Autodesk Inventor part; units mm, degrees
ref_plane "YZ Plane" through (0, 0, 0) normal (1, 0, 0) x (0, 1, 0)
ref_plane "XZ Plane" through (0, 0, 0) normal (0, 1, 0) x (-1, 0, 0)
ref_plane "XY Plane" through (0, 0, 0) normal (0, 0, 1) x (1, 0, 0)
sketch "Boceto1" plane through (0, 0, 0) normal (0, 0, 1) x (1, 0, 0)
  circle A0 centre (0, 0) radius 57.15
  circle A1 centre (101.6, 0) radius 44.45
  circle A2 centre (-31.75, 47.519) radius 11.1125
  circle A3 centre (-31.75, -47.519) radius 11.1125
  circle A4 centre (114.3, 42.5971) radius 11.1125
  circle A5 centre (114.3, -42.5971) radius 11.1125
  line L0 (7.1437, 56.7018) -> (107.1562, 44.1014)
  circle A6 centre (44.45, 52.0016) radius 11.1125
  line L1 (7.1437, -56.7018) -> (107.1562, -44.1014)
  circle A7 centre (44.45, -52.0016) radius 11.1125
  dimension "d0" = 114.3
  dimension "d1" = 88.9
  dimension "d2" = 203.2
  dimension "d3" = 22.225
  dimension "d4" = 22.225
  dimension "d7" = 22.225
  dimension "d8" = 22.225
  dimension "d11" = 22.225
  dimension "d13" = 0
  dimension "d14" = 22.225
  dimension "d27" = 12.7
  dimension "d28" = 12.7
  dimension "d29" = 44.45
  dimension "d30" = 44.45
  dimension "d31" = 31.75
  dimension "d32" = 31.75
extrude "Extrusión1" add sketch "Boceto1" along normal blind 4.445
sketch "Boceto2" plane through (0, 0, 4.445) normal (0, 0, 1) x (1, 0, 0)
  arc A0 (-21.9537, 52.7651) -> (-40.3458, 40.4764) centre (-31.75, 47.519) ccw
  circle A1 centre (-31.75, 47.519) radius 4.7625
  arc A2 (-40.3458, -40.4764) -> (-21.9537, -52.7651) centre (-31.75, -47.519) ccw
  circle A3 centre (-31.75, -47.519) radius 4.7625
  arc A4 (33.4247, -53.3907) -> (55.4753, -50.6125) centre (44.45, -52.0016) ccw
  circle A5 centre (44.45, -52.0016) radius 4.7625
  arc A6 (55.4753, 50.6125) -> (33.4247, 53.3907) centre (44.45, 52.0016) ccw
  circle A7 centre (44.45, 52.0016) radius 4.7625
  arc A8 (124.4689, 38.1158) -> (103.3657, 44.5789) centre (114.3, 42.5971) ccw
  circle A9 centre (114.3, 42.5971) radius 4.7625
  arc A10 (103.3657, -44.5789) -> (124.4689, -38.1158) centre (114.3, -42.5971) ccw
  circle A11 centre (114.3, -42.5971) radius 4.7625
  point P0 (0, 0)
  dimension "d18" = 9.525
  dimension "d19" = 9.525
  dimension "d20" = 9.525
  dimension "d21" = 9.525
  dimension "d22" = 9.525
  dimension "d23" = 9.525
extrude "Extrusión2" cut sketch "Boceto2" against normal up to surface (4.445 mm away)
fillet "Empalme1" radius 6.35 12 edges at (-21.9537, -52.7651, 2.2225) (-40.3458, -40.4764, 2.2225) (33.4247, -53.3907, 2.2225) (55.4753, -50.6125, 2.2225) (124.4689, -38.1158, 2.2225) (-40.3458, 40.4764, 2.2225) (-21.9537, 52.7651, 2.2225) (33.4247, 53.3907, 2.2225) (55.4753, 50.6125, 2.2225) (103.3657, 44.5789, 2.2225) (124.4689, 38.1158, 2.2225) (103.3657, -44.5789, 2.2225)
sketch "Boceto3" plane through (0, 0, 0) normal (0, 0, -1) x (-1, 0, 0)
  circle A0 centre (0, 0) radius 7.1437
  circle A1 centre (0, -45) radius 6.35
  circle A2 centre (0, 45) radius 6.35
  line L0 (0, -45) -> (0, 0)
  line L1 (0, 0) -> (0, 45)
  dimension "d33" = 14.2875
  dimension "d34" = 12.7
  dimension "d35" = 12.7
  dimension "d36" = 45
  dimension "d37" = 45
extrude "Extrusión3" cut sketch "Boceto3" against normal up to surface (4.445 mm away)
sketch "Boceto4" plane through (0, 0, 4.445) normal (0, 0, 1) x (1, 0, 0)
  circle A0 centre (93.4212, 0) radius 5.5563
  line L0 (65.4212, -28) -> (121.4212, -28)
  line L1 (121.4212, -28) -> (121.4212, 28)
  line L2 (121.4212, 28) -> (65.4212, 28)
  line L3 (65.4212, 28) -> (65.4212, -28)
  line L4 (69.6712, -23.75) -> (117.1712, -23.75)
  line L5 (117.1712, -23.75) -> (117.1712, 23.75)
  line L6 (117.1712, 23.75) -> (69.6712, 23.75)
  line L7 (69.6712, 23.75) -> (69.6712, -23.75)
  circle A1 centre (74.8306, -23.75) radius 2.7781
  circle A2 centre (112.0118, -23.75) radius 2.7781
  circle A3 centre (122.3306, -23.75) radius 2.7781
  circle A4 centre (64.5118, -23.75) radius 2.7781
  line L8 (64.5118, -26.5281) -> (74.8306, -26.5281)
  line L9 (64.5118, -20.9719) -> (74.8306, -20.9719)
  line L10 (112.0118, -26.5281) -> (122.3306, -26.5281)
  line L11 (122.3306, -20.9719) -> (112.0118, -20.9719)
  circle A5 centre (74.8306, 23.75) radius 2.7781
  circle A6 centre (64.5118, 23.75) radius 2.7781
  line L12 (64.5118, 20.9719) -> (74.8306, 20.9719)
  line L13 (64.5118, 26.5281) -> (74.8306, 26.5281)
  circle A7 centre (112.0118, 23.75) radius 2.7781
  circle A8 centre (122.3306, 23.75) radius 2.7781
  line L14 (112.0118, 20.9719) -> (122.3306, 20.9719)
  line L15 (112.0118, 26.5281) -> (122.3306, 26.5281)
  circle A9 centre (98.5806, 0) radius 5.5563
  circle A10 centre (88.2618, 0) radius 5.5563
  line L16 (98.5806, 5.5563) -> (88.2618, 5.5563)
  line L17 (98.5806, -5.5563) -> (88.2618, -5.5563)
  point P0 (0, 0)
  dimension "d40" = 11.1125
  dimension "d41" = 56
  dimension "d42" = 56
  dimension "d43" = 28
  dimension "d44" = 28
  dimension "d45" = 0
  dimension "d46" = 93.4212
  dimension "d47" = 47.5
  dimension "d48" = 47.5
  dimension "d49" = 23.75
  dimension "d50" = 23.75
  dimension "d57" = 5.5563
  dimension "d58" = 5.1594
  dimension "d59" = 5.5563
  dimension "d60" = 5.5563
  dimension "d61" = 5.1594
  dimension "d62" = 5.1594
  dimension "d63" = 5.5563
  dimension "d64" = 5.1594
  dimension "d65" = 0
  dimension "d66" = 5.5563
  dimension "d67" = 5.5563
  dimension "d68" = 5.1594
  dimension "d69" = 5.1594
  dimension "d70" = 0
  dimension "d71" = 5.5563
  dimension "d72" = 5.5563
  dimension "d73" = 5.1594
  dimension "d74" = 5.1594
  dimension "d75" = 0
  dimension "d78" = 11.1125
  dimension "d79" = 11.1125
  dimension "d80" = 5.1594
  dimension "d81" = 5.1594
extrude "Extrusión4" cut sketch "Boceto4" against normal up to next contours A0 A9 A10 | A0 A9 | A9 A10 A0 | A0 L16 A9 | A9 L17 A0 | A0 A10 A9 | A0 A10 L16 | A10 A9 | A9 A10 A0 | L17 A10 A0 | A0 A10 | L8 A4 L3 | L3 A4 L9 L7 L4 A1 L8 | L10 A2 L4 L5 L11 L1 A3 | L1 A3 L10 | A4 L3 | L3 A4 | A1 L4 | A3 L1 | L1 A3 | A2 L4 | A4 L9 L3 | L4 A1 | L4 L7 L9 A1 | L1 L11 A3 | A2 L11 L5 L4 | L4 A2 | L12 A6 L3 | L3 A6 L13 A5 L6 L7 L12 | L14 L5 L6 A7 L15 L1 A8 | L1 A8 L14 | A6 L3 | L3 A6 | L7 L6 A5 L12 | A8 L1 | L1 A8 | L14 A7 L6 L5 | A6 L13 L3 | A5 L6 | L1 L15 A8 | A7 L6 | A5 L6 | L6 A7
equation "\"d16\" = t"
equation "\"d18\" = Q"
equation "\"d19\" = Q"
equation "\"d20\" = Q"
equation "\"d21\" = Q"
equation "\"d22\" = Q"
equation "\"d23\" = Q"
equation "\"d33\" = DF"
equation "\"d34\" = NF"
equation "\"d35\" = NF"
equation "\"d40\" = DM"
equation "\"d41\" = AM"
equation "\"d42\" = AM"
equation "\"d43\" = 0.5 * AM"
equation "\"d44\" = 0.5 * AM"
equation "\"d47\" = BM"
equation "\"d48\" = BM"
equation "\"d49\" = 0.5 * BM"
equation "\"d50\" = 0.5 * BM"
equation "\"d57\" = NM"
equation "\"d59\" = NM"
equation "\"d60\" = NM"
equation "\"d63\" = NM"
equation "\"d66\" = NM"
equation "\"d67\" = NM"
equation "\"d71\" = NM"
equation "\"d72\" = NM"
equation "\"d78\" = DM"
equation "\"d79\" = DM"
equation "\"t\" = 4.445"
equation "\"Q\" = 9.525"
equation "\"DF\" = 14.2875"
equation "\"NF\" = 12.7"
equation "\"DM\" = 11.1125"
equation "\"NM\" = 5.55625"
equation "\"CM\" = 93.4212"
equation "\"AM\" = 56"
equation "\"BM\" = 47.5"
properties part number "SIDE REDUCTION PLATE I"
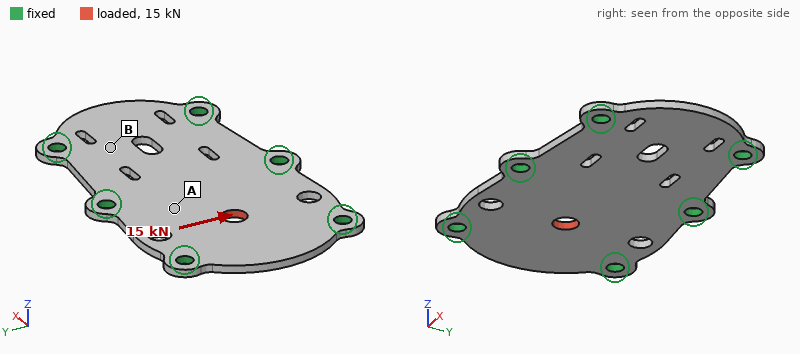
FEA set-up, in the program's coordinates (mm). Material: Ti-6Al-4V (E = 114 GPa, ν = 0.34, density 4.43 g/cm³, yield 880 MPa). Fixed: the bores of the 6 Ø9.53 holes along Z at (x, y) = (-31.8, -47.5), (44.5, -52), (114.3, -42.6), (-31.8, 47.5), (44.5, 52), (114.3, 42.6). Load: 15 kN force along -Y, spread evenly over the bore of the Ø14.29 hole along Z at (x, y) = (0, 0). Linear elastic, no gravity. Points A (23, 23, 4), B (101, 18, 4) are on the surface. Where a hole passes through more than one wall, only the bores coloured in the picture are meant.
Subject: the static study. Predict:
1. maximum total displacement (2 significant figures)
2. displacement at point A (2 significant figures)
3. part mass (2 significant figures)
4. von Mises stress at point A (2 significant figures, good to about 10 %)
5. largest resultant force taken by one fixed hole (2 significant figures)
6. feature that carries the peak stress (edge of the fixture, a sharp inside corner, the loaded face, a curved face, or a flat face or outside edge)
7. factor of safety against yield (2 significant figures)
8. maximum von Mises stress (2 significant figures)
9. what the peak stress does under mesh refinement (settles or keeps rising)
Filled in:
23 µm
9.9 µm
360 g
30 MPa
4.6 kN
the loaded face
6.7
130 MPa
settles
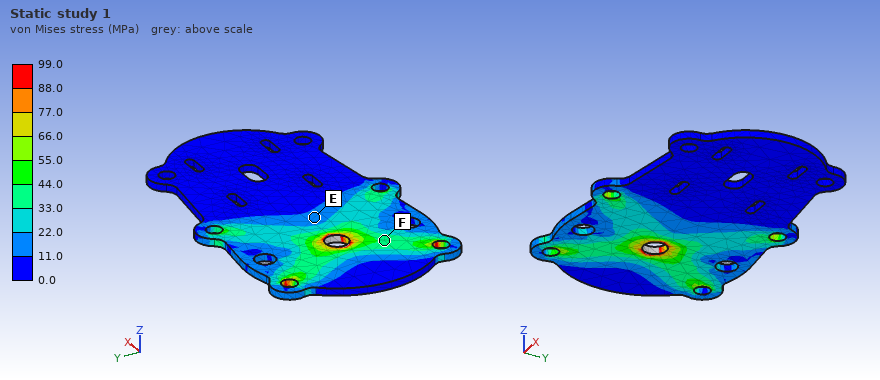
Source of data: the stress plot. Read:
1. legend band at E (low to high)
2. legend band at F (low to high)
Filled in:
11.0 to 22.0 MPa
33.0 to 44.0 MPa
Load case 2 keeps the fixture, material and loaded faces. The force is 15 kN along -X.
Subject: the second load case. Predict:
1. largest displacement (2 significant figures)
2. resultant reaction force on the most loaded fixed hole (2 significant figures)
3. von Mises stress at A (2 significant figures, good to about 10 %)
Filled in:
26 µm
3.5 kN
29 MPa
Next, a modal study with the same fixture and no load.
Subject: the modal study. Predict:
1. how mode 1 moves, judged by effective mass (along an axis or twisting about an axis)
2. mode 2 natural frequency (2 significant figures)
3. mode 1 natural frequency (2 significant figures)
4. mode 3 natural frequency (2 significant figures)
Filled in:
along Z
2500 Hz
2100 Hz
2500 Hz
